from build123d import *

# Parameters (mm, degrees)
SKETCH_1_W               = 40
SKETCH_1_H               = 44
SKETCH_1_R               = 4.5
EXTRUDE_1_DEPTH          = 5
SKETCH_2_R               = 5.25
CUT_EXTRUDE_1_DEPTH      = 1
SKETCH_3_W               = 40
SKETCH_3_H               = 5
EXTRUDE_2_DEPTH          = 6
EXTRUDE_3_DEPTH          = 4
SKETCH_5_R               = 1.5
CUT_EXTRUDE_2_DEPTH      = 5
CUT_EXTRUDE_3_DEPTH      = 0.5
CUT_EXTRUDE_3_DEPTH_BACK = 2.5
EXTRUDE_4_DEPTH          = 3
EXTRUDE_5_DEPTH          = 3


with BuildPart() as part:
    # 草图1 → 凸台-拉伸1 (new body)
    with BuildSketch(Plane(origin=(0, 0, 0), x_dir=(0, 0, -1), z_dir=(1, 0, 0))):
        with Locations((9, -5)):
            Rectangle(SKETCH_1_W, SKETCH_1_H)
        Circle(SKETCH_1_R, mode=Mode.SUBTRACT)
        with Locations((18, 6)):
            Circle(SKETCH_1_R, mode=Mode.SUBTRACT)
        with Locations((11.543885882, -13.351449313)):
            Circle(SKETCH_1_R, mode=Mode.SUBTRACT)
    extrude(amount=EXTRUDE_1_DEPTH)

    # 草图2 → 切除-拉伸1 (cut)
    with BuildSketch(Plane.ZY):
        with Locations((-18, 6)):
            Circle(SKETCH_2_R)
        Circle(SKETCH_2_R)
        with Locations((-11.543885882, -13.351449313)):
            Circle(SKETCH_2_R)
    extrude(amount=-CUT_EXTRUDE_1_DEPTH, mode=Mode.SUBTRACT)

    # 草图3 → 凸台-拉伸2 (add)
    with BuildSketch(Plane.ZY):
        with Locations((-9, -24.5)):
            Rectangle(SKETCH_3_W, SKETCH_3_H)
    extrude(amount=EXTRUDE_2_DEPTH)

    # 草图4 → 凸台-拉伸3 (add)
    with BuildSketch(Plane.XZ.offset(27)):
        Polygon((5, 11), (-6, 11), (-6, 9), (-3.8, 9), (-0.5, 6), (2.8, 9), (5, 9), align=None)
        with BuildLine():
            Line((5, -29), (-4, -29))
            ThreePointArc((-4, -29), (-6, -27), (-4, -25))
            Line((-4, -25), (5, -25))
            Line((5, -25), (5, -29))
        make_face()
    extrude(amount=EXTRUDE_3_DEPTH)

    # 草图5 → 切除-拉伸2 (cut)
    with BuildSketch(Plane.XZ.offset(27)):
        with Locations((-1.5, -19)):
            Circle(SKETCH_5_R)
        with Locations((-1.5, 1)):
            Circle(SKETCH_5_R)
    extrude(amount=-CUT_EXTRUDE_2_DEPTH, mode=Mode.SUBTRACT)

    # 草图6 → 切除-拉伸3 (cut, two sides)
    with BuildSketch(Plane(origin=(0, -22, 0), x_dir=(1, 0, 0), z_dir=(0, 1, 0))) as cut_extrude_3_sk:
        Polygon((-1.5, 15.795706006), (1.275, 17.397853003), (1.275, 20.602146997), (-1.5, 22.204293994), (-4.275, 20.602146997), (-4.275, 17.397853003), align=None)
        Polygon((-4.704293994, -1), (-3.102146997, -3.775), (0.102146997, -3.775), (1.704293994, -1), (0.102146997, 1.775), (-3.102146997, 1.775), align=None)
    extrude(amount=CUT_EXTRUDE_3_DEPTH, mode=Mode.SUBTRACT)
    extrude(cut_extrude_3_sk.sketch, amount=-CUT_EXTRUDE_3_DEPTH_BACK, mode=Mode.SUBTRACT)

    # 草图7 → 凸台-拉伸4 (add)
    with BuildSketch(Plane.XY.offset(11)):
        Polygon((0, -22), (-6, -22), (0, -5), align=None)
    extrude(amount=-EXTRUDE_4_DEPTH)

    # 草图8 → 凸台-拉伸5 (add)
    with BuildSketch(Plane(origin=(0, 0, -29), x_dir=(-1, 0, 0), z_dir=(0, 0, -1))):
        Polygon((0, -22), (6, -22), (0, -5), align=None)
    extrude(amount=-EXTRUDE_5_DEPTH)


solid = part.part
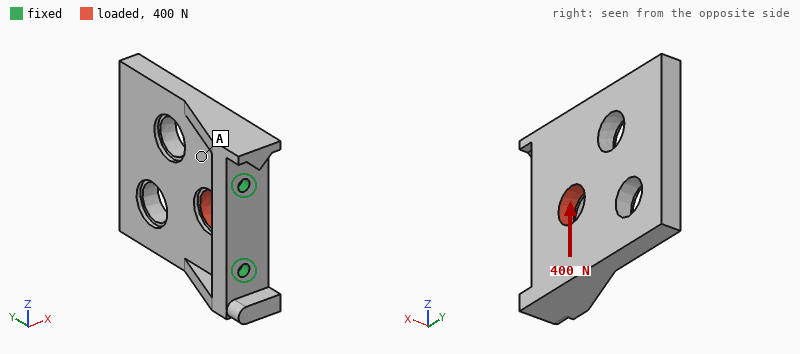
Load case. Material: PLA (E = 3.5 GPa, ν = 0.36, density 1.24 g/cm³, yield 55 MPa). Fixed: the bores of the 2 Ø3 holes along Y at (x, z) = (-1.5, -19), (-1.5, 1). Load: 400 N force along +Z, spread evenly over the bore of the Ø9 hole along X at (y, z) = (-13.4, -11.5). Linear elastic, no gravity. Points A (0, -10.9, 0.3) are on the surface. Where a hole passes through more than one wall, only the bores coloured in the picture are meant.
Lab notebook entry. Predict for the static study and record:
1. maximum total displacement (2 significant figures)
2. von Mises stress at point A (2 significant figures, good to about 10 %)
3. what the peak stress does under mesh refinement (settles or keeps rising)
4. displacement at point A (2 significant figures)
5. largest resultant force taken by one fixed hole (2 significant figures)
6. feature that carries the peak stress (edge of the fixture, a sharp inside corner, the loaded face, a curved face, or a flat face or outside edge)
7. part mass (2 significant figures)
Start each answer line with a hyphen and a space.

- 0.24 mm
- 3.4 MPa
- keeps rising
- 0.11 mm
- 320 N
- edge of the fixture
- 12 g
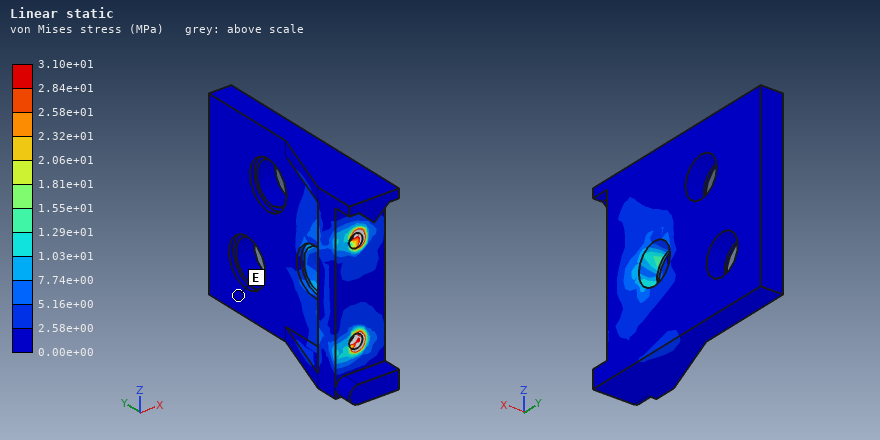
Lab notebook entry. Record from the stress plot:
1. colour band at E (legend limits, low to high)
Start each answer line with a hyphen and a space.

- 0.00e+00 to 2.58e+00 MPa
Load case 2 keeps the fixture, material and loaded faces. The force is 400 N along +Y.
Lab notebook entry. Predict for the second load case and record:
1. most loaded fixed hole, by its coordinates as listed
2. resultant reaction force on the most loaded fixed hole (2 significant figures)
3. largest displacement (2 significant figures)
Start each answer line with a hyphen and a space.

- (-1.5, -19)
- 250 N
- 0.72 mm
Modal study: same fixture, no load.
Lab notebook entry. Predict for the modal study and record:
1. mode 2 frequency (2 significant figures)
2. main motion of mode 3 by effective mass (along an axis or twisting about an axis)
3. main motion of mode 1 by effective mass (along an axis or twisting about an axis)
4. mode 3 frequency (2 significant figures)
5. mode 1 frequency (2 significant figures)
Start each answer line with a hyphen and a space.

- 1400 Hz
- along Z
- along X
- 2000 Hz
- 550 Hz
